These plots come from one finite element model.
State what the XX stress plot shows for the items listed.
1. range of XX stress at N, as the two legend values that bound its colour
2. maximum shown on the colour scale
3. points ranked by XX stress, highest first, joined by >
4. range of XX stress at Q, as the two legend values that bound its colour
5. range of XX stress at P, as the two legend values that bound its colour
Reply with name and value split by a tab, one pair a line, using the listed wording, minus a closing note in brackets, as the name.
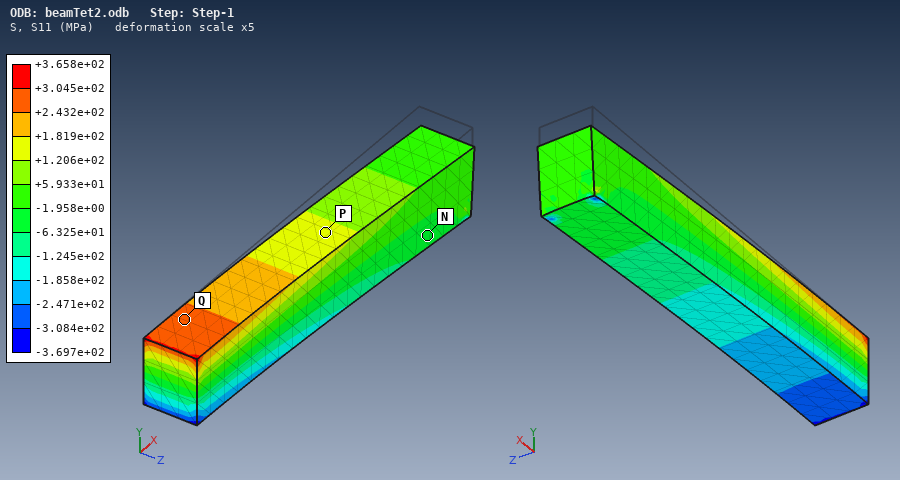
range of XX stress at N, as the two legend values that bound its colour	-6.325e+01 to -1.958e+00 MPa
maximum shown on the colour scale	+3.658e+02 MPa
points ranked by XX stress, highest first, joined by >	Q > P > N
range of XX stress at Q, as the two legend values that bound its colour	+2.432e+02 to +3.045e+02 MPa
range of XX stress at P, as the two legend values that bound its colour	+1.206e+02 to +1.819e+02 MPa
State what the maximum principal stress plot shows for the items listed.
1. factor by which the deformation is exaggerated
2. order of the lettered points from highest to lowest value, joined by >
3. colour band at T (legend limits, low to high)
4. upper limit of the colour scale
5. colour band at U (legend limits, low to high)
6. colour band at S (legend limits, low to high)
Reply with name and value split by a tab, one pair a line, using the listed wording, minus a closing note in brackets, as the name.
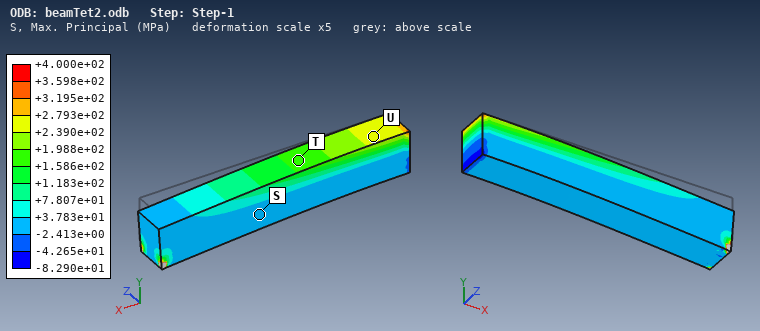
factor by which the deformation is exaggerated	5
order of the lettered points from highest to lowest value, joined by >	U > T > S
colour band at T	+1.586e+02 to +1.988e+02 MPa
upper limit of the colour scale	+4.000e+02 MPa
colour band at U	+2.390e+02 to +2.793e+02 MPa
colour band at S	-2.413e+00 to +3.783e+01 MPa
